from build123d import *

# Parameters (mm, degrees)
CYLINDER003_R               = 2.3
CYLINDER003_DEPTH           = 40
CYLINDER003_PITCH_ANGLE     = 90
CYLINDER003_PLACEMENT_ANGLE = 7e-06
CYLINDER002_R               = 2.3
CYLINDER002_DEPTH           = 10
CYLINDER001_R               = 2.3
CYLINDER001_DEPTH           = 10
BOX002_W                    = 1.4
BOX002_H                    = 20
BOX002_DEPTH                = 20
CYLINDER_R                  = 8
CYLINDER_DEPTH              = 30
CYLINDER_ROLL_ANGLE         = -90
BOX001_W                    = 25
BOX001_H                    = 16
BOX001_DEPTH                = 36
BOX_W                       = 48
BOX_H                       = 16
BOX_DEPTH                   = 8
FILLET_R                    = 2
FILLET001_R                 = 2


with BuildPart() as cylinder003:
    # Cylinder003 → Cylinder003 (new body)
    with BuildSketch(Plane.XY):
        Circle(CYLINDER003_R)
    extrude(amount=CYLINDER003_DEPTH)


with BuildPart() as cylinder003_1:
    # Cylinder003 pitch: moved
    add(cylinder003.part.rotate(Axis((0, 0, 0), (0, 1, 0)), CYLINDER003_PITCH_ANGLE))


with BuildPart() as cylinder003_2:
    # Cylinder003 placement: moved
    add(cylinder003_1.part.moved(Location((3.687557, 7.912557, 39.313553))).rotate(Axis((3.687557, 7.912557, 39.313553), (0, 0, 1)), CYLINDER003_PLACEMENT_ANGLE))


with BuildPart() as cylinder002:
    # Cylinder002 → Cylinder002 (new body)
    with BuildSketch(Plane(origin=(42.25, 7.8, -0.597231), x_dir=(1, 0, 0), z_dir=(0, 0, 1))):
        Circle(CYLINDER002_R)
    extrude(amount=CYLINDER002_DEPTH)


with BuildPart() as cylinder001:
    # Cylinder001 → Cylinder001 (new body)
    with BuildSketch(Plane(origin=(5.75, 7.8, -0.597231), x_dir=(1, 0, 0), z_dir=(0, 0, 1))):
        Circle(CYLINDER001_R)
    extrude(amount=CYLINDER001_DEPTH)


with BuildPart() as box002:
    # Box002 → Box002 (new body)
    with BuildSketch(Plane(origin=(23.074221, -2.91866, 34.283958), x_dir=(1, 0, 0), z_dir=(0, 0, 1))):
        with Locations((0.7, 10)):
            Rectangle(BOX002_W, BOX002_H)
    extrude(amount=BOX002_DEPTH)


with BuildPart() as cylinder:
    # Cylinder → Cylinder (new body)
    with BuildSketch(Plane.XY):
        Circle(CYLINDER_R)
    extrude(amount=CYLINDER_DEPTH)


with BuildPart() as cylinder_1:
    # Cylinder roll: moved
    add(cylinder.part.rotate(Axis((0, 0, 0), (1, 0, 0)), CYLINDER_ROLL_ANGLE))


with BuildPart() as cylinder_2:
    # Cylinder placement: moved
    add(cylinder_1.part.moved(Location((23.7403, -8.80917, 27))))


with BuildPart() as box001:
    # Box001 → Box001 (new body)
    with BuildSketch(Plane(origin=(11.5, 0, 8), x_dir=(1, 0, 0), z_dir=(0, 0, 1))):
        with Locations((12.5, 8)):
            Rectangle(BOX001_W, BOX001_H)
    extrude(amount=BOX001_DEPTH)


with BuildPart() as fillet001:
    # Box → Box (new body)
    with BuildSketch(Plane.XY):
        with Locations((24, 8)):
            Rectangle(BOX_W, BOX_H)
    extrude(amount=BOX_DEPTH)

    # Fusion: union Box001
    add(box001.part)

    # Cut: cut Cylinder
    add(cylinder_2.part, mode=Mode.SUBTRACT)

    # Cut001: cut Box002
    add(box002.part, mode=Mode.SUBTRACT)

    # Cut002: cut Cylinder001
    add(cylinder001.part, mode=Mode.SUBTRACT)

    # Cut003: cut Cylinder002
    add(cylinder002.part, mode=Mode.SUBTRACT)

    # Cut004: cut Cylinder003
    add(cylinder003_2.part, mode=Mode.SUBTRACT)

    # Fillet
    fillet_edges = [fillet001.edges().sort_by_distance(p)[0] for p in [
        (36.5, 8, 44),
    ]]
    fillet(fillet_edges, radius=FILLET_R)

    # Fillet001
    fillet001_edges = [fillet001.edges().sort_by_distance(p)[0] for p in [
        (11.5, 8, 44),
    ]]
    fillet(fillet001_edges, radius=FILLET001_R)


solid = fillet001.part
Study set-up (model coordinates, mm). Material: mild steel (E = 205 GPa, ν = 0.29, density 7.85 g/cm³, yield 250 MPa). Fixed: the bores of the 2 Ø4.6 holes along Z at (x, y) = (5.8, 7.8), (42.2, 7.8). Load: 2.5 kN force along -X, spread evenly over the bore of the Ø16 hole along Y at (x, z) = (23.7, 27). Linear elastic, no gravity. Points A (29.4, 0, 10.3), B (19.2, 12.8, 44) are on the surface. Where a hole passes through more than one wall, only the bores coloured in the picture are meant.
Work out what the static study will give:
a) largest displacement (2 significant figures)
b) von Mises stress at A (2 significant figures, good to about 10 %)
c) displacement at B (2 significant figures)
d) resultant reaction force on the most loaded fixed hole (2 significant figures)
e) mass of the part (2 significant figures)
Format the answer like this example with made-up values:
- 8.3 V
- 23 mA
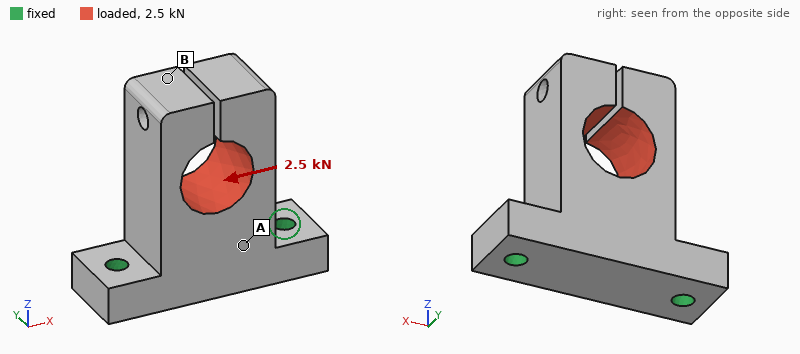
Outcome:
- 50 µm
- 15 MPa
- 48 µm
- 2.3 kN
- 130 g
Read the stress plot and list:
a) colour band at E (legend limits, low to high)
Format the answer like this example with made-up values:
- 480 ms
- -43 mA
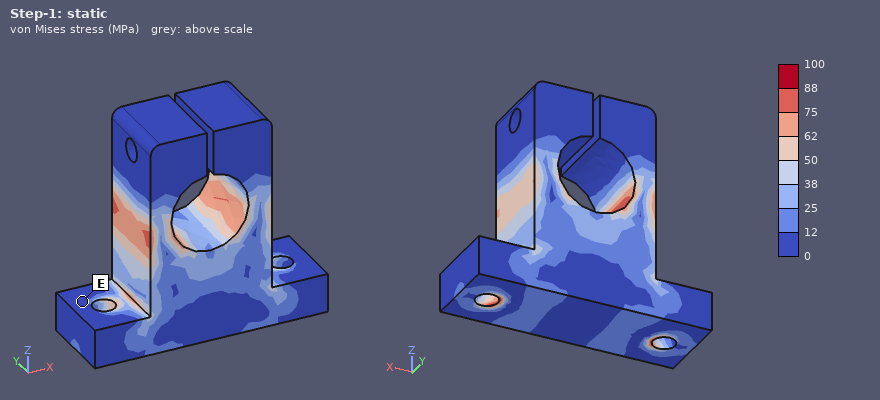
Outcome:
- 0 to 12 MPa
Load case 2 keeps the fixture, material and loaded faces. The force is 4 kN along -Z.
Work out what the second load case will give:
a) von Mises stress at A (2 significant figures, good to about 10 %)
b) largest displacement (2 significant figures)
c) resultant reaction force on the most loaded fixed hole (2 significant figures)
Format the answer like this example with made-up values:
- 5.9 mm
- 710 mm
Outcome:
- 14 MPa
- 44 µm
- 2.2 kN
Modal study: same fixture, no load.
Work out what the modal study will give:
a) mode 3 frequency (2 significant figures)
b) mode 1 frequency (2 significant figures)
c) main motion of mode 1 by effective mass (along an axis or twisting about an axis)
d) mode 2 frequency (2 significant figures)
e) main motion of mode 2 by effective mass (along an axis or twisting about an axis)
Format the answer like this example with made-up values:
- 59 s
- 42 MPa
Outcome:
- 4700 Hz
- 3900 Hz
- along Y
- 4200 Hz
- along X
